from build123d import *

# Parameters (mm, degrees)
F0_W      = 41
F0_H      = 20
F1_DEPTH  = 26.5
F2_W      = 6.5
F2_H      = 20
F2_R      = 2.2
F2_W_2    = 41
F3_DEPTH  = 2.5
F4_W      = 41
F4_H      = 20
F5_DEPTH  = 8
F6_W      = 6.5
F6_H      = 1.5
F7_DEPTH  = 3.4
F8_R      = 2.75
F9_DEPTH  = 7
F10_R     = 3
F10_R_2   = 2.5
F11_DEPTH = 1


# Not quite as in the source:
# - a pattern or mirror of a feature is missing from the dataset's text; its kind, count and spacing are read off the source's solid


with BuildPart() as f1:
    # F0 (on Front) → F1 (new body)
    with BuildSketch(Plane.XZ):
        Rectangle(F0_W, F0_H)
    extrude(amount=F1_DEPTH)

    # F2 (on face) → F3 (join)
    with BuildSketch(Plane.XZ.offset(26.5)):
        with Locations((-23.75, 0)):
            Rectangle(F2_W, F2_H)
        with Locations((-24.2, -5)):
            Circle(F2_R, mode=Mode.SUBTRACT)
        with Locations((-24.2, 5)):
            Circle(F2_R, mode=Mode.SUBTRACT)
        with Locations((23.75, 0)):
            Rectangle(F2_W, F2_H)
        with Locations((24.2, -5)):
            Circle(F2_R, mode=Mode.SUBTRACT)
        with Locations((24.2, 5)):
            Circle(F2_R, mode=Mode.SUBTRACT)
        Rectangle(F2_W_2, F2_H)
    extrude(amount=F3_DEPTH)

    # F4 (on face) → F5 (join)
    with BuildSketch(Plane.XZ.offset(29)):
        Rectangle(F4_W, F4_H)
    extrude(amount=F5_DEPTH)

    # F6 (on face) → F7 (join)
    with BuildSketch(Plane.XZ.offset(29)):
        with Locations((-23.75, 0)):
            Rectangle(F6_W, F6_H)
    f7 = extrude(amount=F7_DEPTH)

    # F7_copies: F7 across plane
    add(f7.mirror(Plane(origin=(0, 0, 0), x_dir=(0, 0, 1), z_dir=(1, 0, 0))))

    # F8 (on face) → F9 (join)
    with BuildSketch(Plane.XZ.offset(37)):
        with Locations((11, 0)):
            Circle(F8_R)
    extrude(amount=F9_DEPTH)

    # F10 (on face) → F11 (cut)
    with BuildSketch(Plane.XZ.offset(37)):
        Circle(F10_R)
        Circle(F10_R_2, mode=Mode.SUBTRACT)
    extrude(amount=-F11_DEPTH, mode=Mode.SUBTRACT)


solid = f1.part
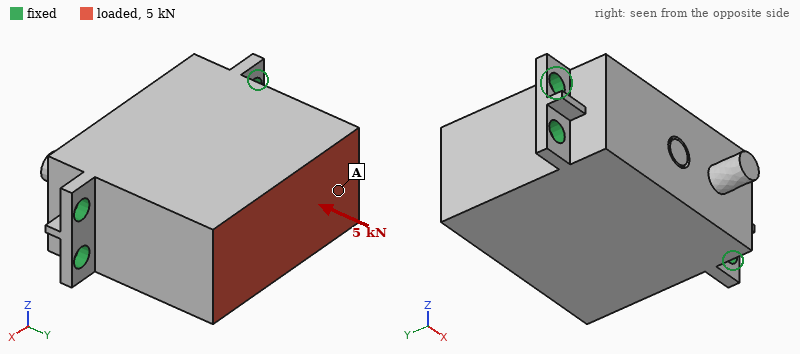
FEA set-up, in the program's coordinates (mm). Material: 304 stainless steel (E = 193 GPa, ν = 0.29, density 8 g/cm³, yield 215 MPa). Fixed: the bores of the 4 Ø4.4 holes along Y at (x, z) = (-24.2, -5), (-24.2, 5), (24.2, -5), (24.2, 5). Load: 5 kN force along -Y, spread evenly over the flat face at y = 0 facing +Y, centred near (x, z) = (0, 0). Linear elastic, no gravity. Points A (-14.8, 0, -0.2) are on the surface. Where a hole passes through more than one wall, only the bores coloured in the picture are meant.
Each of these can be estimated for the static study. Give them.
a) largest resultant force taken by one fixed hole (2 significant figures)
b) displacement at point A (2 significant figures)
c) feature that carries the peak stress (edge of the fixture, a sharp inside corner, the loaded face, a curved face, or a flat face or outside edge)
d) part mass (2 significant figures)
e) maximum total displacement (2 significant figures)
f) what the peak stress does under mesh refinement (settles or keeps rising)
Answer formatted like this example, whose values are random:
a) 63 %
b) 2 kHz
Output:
a) 1.3 kN
b) 5.0 µm
c) edge of the fixture
d) 250 g
e) 5.2 µm
f) keeps rising
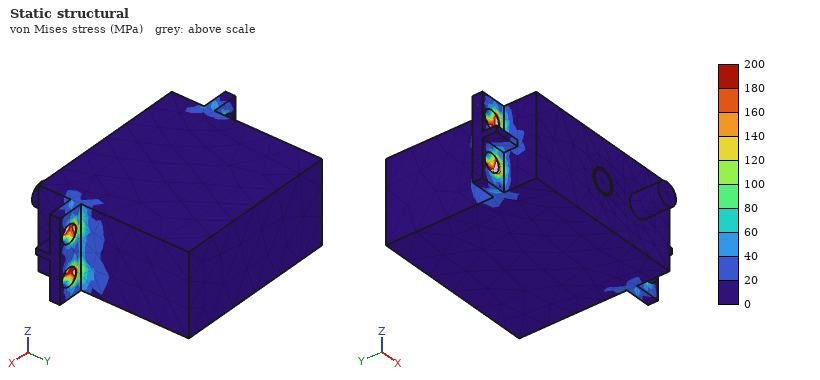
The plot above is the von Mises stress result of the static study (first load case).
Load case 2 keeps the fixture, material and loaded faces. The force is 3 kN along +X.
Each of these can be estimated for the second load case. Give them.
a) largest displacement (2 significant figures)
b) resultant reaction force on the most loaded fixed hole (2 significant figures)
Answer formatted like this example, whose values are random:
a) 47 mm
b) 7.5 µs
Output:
a) 8.0 µm
b) 1.2 kN
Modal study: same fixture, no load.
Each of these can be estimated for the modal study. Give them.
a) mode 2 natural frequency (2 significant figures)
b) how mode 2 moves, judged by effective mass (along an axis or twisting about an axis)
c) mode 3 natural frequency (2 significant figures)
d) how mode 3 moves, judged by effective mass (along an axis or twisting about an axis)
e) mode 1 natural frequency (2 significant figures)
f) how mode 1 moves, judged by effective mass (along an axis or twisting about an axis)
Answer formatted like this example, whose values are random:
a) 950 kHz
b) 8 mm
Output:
a) 11 kHz
b) along Y
c) 11 kHz
d) along X
e) 4000 Hz
f) along Z
